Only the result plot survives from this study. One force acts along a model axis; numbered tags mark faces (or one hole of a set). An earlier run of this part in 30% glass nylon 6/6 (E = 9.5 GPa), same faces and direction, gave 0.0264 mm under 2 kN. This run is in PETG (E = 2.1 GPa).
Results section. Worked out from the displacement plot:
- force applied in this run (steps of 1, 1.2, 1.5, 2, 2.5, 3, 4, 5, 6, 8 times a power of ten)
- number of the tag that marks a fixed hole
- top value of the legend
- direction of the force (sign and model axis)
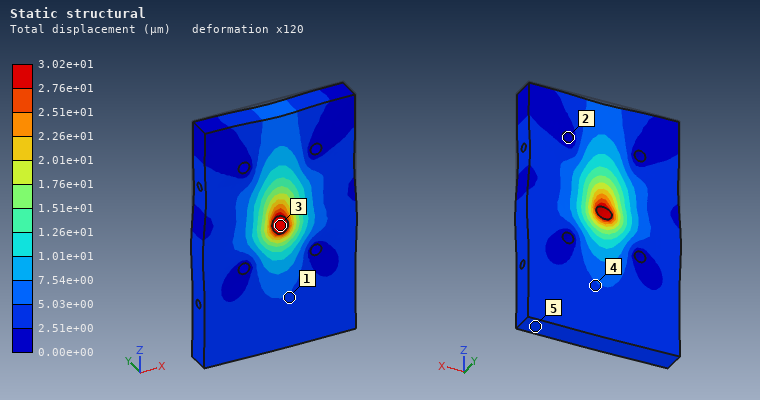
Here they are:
500 N
2
3.02e+01 µm
-Z
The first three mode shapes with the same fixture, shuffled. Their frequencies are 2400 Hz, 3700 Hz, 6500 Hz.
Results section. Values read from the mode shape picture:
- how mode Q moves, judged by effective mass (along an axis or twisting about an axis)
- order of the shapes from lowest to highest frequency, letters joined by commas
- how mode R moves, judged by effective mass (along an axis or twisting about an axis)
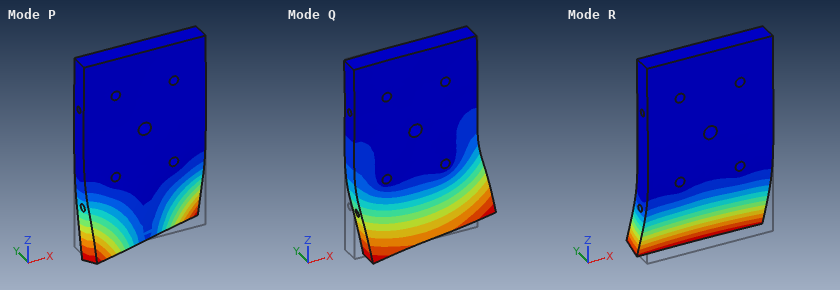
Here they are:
along X
R, P, Q
along Y
